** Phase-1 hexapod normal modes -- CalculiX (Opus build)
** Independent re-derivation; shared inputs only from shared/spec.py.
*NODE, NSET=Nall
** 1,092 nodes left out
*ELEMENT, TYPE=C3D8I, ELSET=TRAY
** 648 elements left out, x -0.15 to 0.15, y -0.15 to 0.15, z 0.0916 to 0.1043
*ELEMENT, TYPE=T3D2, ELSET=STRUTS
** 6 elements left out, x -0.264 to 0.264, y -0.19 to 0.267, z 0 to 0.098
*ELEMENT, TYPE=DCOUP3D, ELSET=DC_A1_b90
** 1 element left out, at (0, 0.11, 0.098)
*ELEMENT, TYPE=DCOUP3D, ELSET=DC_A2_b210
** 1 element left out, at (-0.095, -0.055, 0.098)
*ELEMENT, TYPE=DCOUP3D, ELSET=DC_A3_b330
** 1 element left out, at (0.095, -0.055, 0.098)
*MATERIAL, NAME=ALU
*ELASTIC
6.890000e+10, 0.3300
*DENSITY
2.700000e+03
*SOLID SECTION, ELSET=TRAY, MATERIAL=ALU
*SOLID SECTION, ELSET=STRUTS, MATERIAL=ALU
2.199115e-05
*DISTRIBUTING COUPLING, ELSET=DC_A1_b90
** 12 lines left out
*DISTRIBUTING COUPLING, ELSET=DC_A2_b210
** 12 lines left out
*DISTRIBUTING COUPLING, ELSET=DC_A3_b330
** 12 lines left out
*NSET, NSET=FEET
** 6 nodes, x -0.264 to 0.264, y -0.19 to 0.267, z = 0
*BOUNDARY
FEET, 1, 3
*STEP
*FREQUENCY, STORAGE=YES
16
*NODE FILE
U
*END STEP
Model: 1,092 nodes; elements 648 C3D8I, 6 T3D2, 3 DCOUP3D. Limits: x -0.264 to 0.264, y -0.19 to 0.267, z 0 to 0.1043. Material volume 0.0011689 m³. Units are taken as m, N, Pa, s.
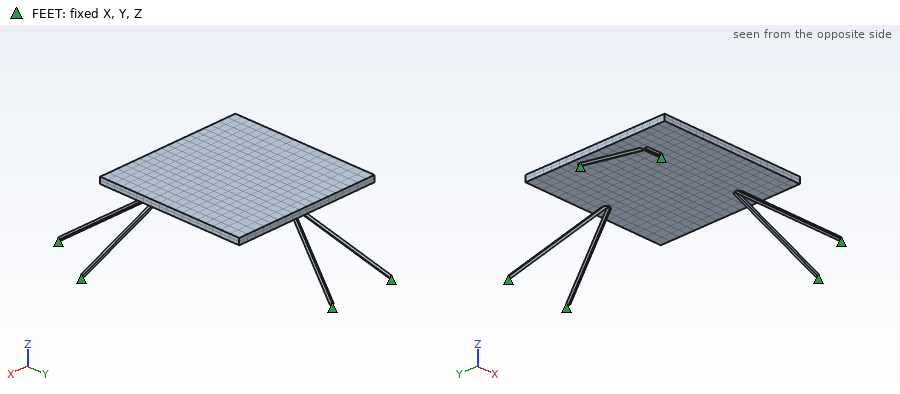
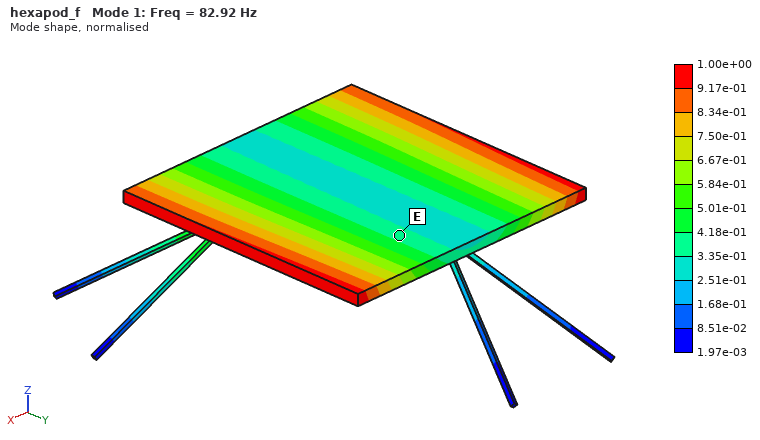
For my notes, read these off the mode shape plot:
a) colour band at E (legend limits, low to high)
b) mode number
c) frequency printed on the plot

3.35e-01 to 4.18e-01
1
82.92 Hz
